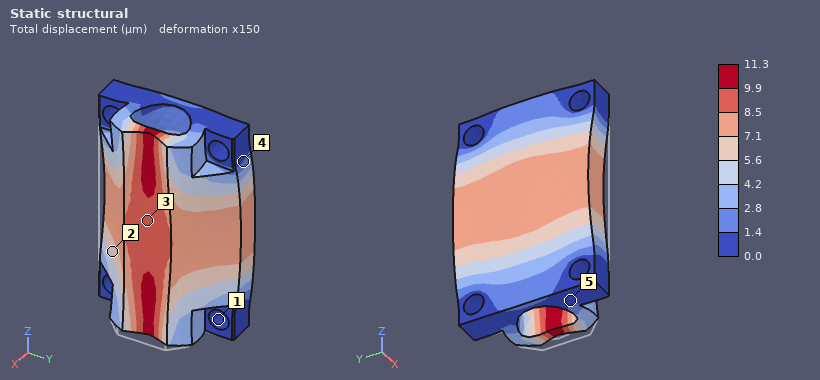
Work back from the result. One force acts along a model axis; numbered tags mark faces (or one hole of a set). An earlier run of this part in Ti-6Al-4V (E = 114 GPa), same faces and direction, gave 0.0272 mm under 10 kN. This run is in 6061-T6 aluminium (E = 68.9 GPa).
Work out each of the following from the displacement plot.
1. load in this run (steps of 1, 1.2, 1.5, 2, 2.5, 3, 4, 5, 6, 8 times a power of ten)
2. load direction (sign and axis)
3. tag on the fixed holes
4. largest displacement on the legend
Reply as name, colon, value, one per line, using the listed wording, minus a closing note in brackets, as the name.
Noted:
load in this run: 2.5 kN
load direction: -X
tag on the fixed holes: 1
largest displacement on the legend: 11.3 µm
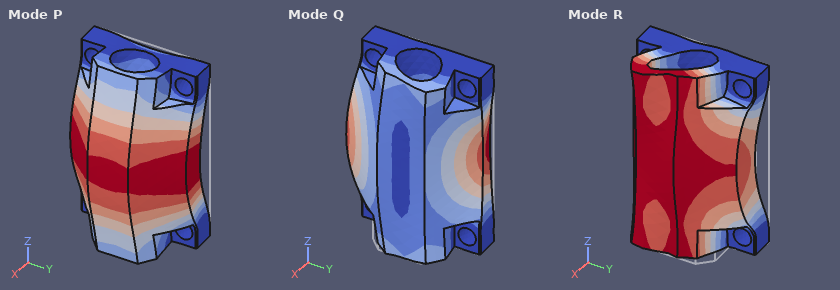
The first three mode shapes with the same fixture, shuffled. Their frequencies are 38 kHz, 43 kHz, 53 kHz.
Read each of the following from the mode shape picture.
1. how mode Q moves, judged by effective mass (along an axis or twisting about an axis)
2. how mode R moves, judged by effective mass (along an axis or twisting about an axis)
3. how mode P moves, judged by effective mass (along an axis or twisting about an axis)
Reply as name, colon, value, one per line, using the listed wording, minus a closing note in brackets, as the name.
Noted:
how mode Q moves, judged by effective mass: along Y
how mode R moves, judged by effective mass: along Y
how mode P moves, judged by effective mass: along X
